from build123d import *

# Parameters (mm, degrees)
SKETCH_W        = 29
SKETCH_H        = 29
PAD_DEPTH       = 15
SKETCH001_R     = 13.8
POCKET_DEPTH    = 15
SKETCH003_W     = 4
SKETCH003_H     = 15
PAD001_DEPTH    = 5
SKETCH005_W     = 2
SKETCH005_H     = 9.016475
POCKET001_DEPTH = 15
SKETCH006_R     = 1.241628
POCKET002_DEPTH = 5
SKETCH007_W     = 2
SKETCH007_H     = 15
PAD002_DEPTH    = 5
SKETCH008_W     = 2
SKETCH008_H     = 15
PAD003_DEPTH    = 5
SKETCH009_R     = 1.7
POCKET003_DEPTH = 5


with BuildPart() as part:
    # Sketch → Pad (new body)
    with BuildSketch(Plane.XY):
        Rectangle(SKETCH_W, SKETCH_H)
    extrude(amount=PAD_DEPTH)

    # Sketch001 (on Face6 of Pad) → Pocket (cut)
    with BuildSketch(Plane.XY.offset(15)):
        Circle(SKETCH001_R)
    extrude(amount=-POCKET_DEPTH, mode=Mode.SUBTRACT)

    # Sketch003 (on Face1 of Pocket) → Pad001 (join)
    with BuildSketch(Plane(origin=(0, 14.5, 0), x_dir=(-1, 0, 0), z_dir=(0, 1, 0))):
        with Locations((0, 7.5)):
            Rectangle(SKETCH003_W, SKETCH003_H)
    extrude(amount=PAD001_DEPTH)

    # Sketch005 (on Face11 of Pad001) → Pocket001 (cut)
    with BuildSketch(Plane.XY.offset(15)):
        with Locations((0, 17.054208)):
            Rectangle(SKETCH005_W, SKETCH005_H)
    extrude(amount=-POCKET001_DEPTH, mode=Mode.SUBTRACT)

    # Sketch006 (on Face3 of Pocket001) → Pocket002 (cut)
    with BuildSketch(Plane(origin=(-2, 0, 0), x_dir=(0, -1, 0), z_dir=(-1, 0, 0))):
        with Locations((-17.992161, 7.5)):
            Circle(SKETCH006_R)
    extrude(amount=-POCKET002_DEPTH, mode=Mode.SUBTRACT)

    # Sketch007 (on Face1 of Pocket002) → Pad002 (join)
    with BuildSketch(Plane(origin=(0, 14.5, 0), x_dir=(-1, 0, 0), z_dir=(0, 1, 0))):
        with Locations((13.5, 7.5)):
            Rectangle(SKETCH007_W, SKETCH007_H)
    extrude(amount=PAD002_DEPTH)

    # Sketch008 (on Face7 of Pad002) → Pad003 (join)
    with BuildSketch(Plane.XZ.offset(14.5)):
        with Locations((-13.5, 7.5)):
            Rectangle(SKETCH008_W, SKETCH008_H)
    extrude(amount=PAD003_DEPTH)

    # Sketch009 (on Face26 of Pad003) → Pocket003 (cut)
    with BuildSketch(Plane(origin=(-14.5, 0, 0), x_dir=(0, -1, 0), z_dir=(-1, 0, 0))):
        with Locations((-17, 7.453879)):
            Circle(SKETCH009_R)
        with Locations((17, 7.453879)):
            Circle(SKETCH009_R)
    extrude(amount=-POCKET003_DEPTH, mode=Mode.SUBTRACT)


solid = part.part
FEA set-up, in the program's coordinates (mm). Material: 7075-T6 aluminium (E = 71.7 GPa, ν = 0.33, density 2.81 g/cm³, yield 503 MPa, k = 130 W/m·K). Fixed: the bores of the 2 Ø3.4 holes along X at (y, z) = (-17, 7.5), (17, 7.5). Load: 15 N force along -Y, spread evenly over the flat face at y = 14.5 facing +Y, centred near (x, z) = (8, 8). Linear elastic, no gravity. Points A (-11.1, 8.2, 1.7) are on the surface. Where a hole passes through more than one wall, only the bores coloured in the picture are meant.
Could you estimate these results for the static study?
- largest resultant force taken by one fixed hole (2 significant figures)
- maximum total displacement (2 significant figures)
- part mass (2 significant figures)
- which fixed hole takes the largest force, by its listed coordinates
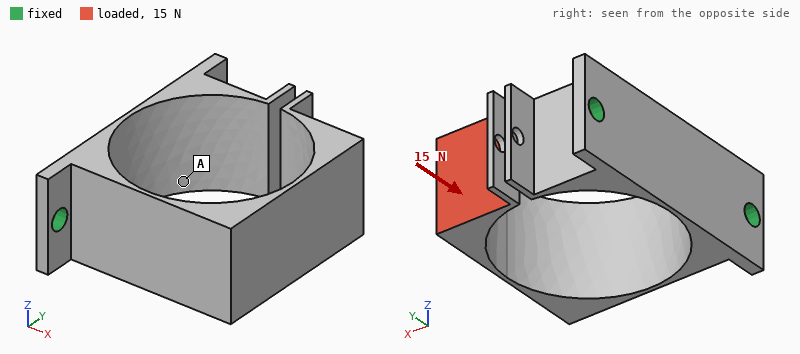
41 N
0.48 mm
11 g
(-17, 7.5)
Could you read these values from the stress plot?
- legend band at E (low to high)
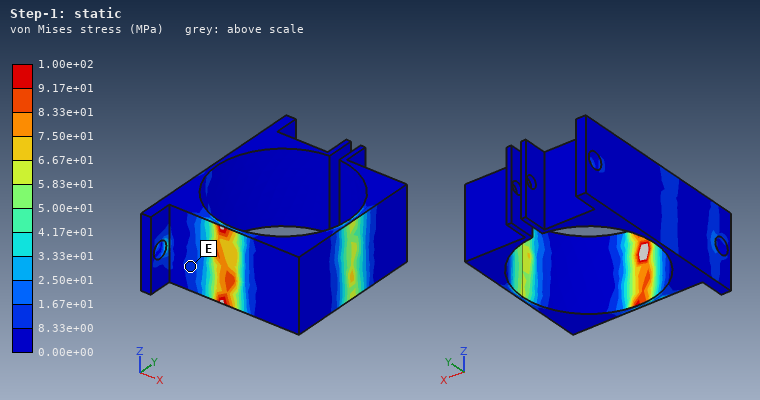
8.33e+00 to 1.67e+01 MPa
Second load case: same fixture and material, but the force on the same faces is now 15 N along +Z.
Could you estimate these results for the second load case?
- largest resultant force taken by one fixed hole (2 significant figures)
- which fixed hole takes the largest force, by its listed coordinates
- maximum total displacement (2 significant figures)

12 N
(17, 7.5)
0.60 mm
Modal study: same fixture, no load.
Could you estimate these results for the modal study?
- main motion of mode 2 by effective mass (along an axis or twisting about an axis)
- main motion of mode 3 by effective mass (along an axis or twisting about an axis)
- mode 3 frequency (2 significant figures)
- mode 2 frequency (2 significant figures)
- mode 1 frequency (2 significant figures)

along Z
along Y
810 Hz
580 Hz
250 Hz
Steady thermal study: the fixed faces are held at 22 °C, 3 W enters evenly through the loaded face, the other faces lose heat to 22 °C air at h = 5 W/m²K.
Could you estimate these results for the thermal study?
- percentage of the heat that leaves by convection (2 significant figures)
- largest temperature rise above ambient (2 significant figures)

11 %
49 K
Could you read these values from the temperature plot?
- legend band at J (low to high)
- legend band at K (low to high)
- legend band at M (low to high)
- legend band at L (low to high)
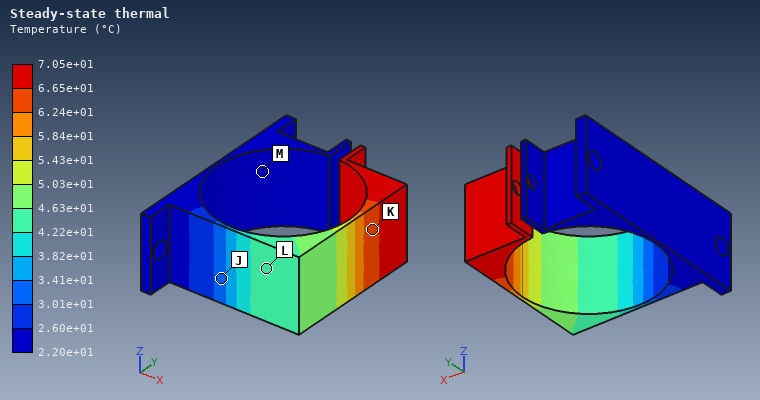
3.01e+01 to 3.41e+01 °C
6.24e+01 to 6.65e+01 °C
2.20e+01 to 2.60e+01 °C
4.22e+01 to 4.63e+01 °C
